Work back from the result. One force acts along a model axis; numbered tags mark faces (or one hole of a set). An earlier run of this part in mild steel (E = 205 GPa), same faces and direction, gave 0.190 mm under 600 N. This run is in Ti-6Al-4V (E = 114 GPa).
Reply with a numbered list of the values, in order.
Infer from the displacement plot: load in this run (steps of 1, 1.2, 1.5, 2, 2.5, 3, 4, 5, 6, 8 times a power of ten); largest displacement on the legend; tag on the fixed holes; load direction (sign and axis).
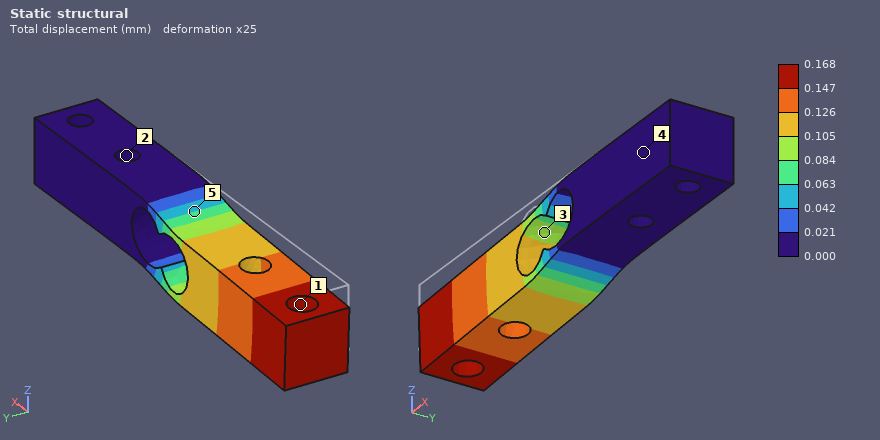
1. 300 N
2. 0.168 mm
3. 2
4. -Z
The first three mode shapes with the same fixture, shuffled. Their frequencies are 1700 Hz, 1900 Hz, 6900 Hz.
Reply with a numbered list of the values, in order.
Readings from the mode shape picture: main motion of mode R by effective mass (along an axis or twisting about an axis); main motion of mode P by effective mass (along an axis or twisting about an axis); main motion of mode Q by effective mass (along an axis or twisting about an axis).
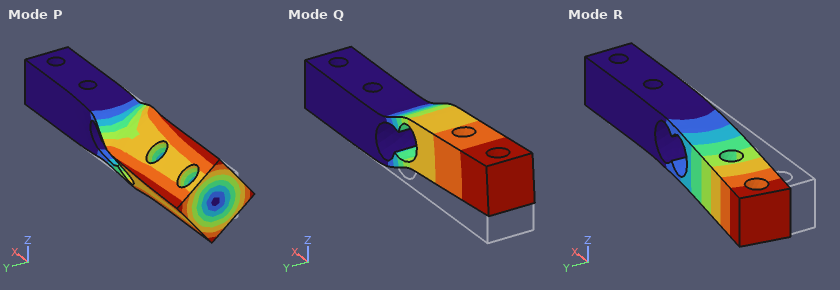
1. along Y
2. twisting about X
3. along Z
